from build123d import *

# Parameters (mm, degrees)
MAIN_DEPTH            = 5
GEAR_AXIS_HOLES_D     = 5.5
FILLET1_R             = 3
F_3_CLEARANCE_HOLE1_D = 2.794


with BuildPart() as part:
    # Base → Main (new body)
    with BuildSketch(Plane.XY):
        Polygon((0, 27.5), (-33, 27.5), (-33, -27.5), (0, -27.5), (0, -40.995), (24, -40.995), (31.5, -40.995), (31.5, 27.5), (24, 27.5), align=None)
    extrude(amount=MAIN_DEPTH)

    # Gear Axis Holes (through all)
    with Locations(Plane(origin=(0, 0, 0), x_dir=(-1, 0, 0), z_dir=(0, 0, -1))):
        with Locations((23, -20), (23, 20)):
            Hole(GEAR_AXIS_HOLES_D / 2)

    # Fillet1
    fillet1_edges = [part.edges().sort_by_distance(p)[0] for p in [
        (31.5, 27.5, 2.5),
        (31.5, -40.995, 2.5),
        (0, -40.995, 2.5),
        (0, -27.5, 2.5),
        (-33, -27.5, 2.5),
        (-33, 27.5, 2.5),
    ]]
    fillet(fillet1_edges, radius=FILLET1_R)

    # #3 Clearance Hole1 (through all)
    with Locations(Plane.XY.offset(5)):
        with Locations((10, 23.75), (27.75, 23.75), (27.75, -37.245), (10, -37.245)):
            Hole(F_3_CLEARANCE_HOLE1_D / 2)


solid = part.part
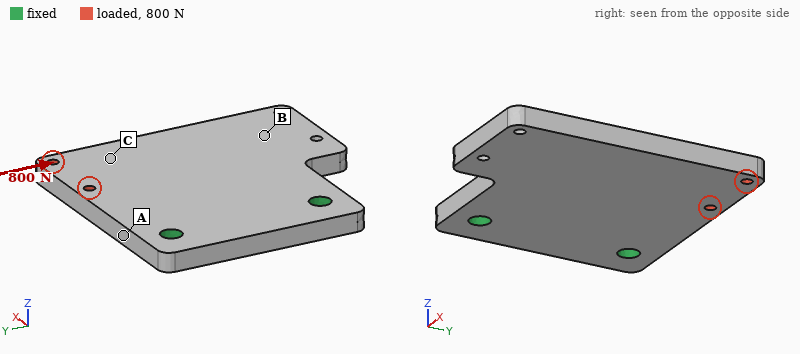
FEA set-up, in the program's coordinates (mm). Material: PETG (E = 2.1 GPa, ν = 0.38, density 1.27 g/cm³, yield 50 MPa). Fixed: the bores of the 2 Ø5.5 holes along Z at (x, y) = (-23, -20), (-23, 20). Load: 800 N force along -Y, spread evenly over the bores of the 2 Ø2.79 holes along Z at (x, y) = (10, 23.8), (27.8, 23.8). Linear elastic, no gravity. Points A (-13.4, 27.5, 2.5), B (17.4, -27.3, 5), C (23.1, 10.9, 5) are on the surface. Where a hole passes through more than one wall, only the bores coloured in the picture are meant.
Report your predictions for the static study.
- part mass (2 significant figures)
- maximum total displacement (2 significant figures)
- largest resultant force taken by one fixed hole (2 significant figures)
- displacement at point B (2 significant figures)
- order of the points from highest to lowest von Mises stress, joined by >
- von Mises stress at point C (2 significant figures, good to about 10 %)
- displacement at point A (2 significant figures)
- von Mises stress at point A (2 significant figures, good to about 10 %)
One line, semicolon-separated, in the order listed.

25 g; 0.51 mm; 890 N; 0.32 mm; A > C > B; 5.4 MPa; 0.11 mm; 9.3 MPa
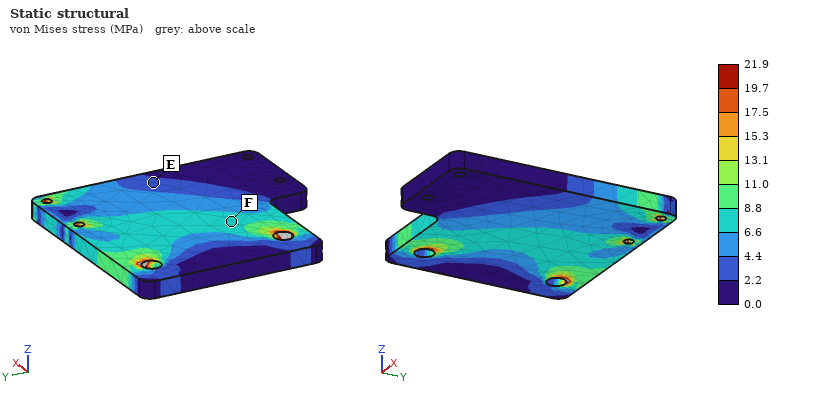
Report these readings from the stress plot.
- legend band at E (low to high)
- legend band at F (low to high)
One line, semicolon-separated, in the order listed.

2.2 to 4.4 MPa; 6.6 to 8.8 MPa
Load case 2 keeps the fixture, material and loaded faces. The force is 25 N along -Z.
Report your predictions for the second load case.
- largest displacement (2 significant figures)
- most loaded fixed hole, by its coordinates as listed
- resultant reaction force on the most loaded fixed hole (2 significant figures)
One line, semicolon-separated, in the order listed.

1.0 mm; (-23, 20); 27 N
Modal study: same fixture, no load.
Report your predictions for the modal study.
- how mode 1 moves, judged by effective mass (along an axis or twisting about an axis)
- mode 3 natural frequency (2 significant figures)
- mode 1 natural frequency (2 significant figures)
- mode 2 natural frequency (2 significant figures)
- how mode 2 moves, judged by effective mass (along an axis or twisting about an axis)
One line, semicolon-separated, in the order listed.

along Z; 1700 Hz; 310 Hz; 630 Hz; twisting about X
